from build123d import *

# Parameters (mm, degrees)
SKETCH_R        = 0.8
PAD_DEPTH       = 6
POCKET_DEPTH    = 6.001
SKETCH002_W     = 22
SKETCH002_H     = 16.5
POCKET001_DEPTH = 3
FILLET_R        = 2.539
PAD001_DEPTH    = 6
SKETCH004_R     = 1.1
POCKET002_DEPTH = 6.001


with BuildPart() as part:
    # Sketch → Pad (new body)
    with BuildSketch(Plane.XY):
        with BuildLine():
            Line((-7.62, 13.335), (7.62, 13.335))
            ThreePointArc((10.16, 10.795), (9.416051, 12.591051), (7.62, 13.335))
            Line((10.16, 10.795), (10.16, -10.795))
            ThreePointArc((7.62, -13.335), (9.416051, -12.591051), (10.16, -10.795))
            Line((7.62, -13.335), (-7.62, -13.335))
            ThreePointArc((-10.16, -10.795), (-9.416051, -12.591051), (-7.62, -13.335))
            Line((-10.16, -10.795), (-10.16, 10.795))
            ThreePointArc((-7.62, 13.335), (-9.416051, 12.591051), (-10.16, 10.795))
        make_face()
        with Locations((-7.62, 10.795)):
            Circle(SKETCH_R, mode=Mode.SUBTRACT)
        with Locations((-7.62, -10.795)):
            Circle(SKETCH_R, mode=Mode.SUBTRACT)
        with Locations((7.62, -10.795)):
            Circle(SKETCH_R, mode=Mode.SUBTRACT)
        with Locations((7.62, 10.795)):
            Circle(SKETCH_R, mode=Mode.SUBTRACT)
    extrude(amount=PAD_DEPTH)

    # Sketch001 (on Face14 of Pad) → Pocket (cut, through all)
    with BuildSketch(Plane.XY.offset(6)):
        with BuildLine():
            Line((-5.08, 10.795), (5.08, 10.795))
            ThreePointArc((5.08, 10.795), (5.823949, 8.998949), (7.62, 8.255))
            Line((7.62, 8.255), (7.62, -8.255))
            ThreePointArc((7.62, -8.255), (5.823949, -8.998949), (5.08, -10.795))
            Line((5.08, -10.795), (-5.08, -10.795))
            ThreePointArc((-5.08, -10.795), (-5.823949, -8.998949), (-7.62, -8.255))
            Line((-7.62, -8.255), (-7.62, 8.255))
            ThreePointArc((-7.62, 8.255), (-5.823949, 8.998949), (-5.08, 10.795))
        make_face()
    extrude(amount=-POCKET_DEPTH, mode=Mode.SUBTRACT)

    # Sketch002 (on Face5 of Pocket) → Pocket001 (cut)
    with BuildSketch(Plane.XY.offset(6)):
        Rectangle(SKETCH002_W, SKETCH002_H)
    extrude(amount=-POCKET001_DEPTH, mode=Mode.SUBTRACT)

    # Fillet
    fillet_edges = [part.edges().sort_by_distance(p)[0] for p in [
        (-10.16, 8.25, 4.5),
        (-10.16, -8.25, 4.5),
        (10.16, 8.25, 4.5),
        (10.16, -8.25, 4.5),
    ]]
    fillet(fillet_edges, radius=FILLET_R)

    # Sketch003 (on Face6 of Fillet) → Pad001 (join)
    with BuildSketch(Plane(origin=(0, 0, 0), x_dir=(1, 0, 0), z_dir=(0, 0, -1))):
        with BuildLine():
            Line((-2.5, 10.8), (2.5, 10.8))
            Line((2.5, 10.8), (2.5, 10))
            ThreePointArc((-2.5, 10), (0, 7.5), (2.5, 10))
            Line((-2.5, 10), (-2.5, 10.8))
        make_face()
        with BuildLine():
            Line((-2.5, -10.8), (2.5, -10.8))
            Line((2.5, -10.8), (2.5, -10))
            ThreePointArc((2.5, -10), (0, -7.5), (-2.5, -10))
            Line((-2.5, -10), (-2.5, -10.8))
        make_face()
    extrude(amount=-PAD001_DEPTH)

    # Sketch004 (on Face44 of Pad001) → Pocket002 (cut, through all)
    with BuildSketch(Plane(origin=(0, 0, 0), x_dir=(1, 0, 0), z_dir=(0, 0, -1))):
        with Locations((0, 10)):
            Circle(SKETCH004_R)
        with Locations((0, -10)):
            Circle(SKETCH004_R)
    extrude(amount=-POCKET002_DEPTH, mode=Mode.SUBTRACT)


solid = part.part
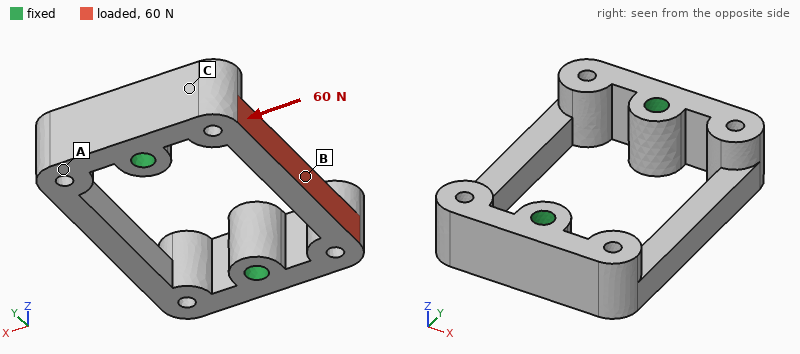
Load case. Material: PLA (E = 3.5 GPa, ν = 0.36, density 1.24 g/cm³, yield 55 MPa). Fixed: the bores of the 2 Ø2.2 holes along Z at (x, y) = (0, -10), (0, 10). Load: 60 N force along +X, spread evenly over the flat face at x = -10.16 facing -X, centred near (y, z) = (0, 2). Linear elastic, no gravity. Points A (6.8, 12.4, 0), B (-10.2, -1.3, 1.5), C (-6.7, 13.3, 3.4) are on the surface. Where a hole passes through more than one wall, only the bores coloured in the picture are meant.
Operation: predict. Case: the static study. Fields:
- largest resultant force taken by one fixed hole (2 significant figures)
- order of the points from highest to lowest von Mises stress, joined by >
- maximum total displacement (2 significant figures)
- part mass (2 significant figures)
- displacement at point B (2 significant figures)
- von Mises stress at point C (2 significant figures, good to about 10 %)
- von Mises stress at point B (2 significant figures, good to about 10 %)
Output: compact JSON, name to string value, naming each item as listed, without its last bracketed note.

{"largest resultant force taken by one fixed hole": "38 N", "order of the points from highest to lowest von Mises stress, joined by >": "B > C > A", "maximum total displacement": "0.13 mm", "part mass": "1.5 g", "displacement at point B": "0.12 mm", "von Mises stress at point C": "3.9 MPa", "von Mises stress at point B": "17 MPa"}
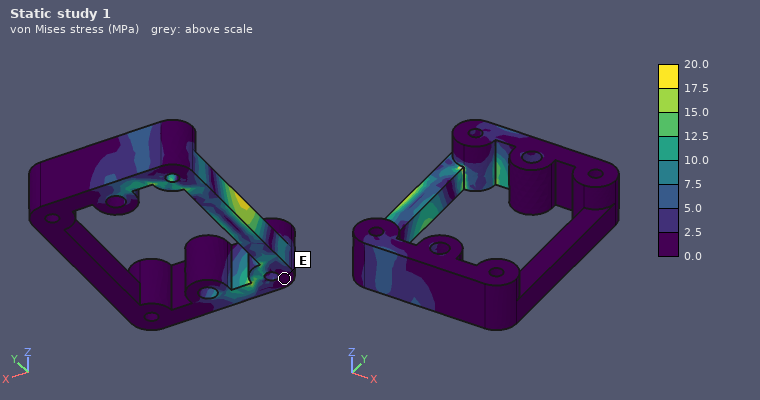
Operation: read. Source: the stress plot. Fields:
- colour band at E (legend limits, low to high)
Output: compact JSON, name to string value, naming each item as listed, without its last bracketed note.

{"colour band at E": "0.0 to 2.5 MPa"}
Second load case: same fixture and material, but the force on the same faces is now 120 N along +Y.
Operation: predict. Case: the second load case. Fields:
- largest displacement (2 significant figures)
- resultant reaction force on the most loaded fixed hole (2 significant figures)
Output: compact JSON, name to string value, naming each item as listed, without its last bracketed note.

{"largest displacement": "0.22 mm", "resultant reaction force on the most loaded fixed hole": "64 N"}
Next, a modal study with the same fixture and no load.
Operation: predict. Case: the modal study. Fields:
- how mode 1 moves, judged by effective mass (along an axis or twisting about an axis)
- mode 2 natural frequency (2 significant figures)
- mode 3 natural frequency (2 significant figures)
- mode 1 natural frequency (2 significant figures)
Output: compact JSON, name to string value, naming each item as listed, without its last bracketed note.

{"how mode 1 moves, judged by effective mass": "twisting about Y", "mode 2 natural frequency": "5900 Hz", "mode 3 natural frequency": "6000 Hz", "mode 1 natural frequency": "5500 Hz"}
